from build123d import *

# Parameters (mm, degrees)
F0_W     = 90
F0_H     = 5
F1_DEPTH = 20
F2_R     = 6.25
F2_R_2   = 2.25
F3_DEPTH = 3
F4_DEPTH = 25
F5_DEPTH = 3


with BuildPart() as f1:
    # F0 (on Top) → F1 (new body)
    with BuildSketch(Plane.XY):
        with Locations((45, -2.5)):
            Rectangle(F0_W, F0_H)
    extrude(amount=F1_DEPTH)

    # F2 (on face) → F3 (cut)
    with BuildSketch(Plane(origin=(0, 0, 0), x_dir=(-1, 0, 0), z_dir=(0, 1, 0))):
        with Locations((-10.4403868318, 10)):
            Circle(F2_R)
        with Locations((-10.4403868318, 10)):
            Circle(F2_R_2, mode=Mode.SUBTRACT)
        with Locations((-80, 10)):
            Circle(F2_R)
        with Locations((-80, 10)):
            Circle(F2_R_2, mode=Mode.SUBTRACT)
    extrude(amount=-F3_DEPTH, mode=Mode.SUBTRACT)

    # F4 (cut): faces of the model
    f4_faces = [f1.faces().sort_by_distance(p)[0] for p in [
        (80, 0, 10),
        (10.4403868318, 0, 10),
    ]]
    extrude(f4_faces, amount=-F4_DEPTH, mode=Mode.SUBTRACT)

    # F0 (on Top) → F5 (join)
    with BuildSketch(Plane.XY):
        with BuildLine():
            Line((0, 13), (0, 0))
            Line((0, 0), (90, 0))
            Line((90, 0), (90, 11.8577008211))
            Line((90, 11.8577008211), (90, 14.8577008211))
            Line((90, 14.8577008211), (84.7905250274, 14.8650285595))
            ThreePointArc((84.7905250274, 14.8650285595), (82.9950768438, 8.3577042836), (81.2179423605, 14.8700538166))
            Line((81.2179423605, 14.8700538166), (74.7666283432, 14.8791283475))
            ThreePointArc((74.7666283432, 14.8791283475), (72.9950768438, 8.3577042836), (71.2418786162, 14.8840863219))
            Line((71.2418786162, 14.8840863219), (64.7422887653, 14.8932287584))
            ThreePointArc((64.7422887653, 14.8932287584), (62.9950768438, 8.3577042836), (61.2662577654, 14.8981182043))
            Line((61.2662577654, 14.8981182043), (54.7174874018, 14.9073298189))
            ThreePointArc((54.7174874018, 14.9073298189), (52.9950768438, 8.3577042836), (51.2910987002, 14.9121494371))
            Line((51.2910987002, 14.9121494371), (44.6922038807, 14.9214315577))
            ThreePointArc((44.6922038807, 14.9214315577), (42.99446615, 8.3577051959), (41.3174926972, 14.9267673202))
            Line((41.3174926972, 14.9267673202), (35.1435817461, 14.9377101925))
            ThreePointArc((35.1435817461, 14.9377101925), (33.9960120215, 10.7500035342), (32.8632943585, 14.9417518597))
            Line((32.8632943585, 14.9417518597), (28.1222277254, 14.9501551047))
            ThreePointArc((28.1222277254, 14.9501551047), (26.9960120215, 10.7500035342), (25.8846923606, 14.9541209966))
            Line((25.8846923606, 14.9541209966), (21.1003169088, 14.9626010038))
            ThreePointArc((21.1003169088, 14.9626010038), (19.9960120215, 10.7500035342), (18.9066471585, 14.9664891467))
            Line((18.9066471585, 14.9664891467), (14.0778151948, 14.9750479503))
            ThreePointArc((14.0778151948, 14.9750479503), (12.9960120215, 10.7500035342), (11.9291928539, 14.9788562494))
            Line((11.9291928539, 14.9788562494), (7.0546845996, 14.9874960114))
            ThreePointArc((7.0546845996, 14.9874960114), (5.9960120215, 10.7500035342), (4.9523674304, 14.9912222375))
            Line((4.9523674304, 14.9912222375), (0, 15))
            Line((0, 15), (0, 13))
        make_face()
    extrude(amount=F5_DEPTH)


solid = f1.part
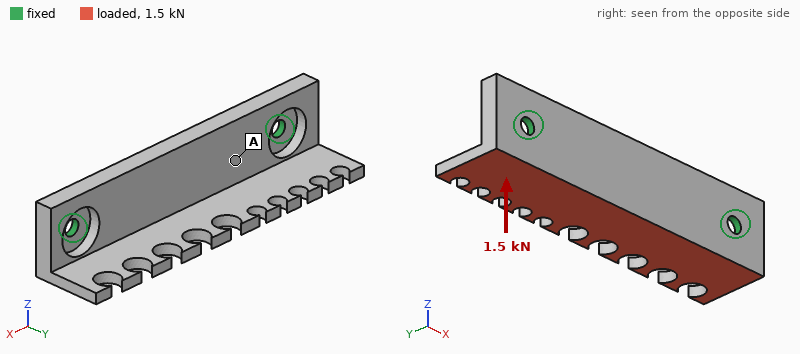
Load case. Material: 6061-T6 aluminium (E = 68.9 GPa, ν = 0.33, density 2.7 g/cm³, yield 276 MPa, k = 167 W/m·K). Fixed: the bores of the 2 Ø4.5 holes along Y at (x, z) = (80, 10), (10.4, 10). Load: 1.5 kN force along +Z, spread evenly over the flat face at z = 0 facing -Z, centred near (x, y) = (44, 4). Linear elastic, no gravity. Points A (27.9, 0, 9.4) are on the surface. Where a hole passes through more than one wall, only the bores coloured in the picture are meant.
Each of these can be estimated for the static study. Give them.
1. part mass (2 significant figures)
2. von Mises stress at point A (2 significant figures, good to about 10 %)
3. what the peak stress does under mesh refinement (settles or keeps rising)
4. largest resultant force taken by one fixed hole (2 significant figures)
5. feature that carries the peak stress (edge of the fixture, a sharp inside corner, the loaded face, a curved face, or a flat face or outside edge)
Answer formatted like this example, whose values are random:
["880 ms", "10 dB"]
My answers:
["31 g", "32 MPa", "keeps rising", "780 N", "edge of the fixture"]
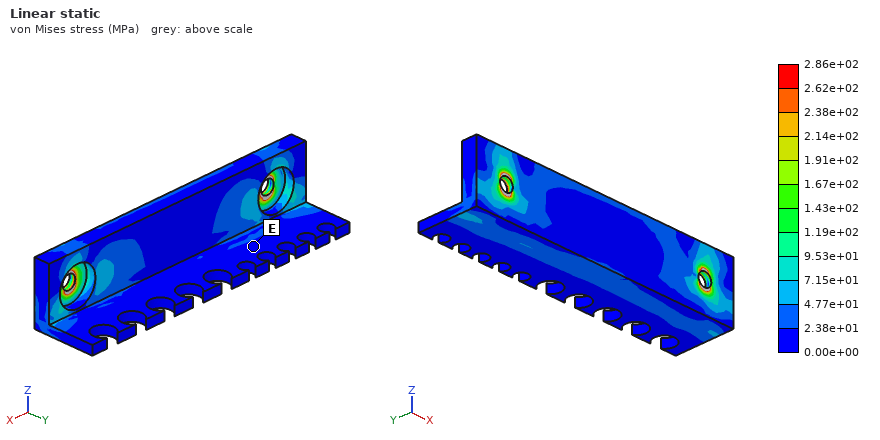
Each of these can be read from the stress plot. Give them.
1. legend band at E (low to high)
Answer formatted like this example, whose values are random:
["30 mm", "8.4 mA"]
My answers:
["0.00e+00 to 2.38e+01 MPa"]
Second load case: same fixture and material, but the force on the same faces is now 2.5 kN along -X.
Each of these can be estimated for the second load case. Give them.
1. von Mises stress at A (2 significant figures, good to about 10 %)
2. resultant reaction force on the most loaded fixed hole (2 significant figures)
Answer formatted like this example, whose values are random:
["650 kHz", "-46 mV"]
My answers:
["11 MPa", "1.3 kN"]
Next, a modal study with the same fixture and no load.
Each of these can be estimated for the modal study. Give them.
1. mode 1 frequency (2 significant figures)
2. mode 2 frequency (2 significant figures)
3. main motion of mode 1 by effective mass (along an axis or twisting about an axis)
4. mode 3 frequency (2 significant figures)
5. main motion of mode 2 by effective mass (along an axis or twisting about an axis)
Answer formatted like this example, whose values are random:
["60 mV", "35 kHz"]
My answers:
["3600 Hz", "5100 Hz", "along Z", "6300 Hz", "along Y"]
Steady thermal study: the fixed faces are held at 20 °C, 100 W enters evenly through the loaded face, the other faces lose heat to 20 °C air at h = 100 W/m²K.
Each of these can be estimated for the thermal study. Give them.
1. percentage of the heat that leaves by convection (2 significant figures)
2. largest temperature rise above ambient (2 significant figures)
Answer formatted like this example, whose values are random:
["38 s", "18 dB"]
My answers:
["21 %", "58 K"]
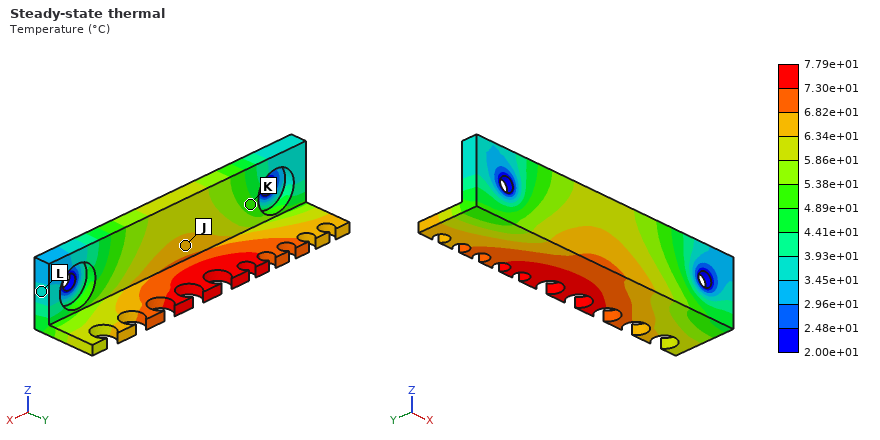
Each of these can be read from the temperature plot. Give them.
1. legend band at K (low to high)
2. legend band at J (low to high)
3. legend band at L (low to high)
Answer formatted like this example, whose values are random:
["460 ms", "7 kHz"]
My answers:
["4.89e+01 to 5.38e+01 °C", "6.34e+01 to 6.82e+01 °C", "3.45e+01 to 3.93e+01 °C"]
